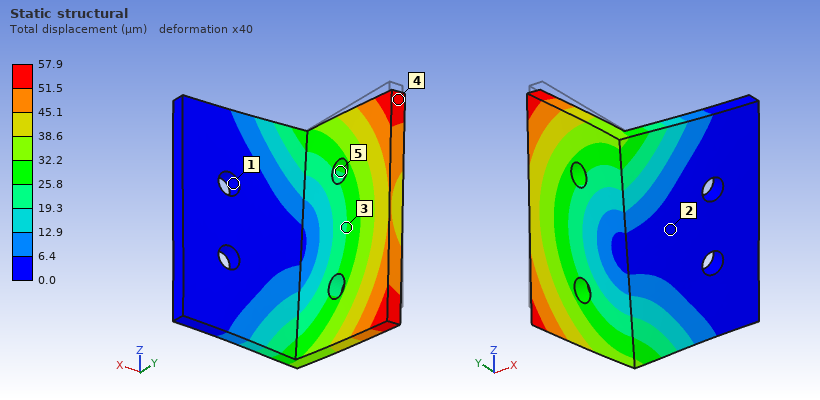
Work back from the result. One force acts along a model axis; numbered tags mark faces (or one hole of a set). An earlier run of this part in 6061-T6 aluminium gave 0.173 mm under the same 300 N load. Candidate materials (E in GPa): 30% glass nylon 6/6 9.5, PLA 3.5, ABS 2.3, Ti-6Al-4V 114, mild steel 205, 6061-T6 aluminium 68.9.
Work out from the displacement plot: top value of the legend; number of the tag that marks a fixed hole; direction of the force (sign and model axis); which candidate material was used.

57.9 µm
1
-Z
mild steel
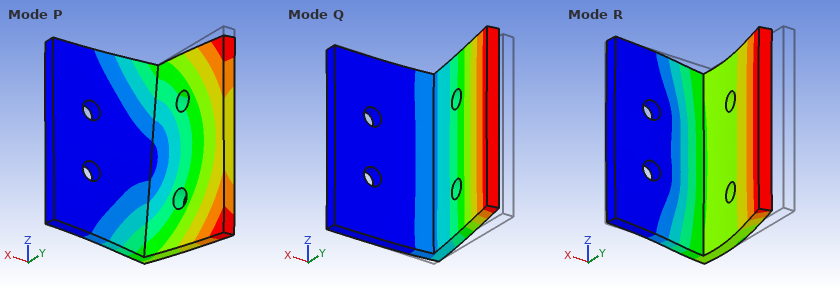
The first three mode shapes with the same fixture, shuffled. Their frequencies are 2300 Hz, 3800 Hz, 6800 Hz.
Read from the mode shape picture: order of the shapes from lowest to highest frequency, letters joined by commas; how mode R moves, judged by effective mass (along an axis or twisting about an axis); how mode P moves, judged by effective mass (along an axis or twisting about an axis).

Q, P, R
along Y
along Z
